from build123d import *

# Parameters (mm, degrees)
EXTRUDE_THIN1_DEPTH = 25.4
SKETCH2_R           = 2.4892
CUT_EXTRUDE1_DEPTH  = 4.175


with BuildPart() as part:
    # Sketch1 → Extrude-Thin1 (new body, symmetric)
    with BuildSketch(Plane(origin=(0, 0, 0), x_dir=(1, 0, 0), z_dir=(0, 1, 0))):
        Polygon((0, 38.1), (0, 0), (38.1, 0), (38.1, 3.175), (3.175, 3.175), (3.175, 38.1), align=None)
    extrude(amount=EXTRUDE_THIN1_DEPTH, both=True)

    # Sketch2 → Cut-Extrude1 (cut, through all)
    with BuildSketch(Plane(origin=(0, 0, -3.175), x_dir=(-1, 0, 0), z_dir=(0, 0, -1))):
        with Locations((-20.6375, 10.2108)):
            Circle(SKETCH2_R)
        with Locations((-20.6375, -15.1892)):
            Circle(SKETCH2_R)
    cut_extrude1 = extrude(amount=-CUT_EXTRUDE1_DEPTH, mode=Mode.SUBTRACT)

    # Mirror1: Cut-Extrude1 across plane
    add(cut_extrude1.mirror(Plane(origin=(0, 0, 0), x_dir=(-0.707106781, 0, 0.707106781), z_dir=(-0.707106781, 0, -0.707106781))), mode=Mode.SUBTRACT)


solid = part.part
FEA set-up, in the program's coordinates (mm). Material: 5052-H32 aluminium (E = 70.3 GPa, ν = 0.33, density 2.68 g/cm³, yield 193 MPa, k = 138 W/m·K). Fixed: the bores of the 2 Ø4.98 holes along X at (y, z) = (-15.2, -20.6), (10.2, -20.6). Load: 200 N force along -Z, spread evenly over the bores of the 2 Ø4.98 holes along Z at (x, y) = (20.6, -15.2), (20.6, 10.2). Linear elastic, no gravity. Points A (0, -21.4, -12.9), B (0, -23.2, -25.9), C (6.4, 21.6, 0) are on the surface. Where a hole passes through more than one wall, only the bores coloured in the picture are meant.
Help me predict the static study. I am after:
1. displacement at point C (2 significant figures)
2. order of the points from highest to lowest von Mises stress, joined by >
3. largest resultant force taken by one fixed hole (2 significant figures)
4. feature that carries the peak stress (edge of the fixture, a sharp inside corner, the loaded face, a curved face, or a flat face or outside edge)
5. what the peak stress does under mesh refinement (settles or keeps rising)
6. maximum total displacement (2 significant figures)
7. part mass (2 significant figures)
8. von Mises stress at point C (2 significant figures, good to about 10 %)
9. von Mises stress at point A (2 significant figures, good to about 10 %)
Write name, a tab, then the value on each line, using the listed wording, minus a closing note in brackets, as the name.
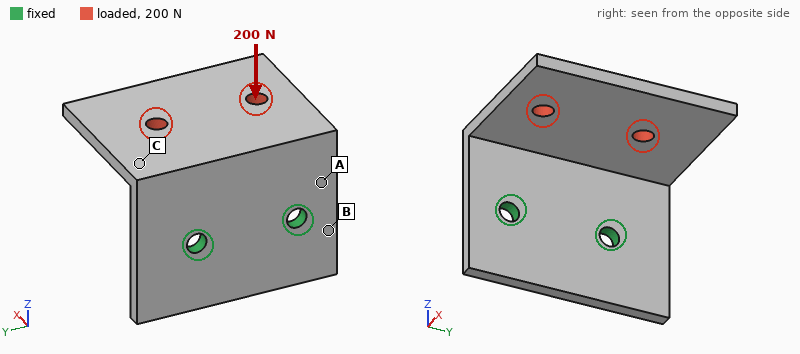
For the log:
displacement at point C	0.085 mm
order of the points from highest to lowest von Mises stress, joined by >	A > C > B
largest resultant force taken by one fixed hole	100 N
feature that carries the peak stress	edge of the fixture
what the peak stress does under mesh refinement	keeps rising
maximum total displacement	0.37 mm
part mass	31 g
von Mises stress at point C	28 MPa
von Mises stress at point A	43 MPa
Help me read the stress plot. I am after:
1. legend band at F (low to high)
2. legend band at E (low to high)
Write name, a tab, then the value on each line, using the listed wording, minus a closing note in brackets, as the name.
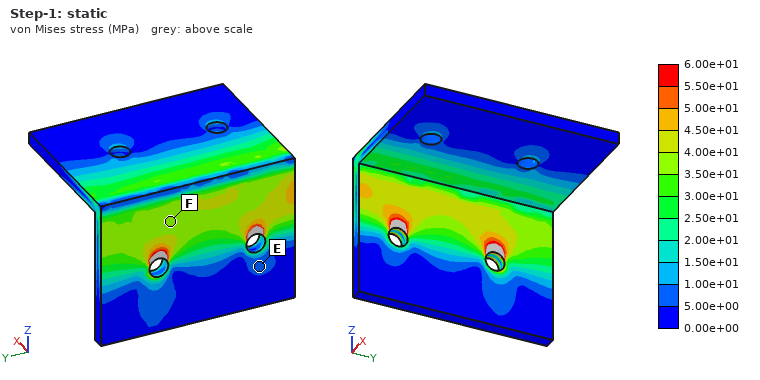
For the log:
legend band at F	3.50e+01 to 4.00e+01 MPa
legend band at E	5.00e+00 to 1.00e+01 MPa
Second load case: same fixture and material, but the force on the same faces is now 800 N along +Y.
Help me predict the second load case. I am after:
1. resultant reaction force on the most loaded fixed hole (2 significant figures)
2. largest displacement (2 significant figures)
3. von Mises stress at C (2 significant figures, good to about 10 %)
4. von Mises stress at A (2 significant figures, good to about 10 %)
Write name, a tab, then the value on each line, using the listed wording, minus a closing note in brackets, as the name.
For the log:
resultant reaction force on the most loaded fixed hole	820 N
largest displacement	0.34 mm
von Mises stress at C	41 MPa
von Mises stress at A	69 MPa
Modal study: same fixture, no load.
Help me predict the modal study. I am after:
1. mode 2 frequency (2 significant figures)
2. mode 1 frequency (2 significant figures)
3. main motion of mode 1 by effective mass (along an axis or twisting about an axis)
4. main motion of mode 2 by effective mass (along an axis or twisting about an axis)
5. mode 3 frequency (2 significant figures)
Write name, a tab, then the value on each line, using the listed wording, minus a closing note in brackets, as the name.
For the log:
mode 2 frequency	2200 Hz
mode 1 frequency	1100 Hz
main motion of mode 1 by effective mass	along Z
main motion of mode 2 by effective mass	along Y
mode 3 frequency	3500 Hz
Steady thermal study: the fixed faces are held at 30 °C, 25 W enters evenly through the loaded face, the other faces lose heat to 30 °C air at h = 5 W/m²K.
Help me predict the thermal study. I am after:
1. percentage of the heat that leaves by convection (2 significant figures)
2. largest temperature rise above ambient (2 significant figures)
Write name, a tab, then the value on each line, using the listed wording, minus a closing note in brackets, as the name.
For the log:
percentage of the heat that leaves by convection	3.6 %
largest temperature rise above ambient	48 K
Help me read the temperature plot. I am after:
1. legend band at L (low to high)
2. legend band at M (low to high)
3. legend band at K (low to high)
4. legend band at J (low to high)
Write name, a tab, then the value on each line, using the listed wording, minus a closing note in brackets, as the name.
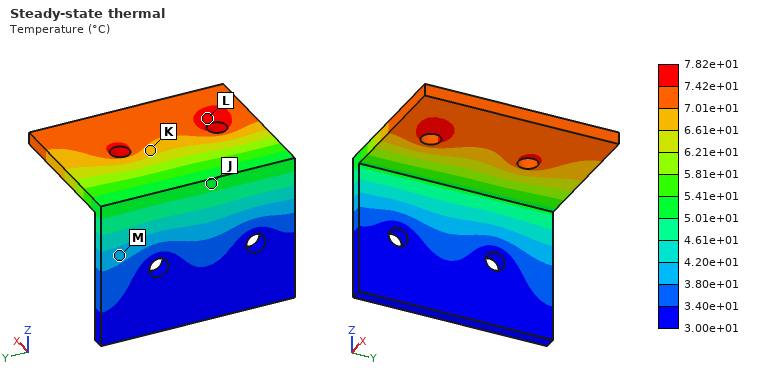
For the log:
legend band at L	7.42e+01 to 7.82e+01 °C
legend band at M	3.80e+01 to 4.20e+01 °C
legend band at K	6.61e+01 to 7.01e+01 °C
legend band at J	5.01e+01 to 5.41e+01 °C
